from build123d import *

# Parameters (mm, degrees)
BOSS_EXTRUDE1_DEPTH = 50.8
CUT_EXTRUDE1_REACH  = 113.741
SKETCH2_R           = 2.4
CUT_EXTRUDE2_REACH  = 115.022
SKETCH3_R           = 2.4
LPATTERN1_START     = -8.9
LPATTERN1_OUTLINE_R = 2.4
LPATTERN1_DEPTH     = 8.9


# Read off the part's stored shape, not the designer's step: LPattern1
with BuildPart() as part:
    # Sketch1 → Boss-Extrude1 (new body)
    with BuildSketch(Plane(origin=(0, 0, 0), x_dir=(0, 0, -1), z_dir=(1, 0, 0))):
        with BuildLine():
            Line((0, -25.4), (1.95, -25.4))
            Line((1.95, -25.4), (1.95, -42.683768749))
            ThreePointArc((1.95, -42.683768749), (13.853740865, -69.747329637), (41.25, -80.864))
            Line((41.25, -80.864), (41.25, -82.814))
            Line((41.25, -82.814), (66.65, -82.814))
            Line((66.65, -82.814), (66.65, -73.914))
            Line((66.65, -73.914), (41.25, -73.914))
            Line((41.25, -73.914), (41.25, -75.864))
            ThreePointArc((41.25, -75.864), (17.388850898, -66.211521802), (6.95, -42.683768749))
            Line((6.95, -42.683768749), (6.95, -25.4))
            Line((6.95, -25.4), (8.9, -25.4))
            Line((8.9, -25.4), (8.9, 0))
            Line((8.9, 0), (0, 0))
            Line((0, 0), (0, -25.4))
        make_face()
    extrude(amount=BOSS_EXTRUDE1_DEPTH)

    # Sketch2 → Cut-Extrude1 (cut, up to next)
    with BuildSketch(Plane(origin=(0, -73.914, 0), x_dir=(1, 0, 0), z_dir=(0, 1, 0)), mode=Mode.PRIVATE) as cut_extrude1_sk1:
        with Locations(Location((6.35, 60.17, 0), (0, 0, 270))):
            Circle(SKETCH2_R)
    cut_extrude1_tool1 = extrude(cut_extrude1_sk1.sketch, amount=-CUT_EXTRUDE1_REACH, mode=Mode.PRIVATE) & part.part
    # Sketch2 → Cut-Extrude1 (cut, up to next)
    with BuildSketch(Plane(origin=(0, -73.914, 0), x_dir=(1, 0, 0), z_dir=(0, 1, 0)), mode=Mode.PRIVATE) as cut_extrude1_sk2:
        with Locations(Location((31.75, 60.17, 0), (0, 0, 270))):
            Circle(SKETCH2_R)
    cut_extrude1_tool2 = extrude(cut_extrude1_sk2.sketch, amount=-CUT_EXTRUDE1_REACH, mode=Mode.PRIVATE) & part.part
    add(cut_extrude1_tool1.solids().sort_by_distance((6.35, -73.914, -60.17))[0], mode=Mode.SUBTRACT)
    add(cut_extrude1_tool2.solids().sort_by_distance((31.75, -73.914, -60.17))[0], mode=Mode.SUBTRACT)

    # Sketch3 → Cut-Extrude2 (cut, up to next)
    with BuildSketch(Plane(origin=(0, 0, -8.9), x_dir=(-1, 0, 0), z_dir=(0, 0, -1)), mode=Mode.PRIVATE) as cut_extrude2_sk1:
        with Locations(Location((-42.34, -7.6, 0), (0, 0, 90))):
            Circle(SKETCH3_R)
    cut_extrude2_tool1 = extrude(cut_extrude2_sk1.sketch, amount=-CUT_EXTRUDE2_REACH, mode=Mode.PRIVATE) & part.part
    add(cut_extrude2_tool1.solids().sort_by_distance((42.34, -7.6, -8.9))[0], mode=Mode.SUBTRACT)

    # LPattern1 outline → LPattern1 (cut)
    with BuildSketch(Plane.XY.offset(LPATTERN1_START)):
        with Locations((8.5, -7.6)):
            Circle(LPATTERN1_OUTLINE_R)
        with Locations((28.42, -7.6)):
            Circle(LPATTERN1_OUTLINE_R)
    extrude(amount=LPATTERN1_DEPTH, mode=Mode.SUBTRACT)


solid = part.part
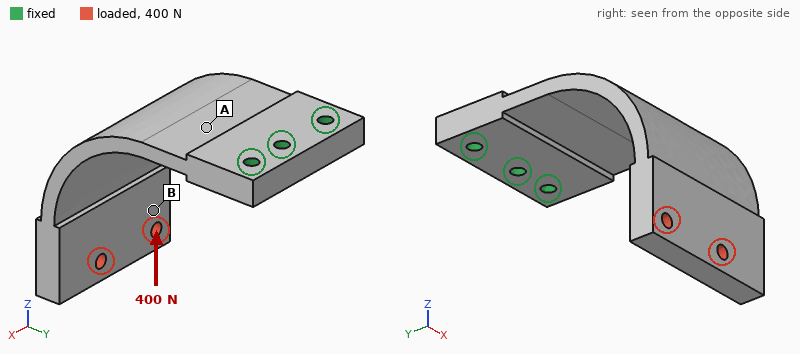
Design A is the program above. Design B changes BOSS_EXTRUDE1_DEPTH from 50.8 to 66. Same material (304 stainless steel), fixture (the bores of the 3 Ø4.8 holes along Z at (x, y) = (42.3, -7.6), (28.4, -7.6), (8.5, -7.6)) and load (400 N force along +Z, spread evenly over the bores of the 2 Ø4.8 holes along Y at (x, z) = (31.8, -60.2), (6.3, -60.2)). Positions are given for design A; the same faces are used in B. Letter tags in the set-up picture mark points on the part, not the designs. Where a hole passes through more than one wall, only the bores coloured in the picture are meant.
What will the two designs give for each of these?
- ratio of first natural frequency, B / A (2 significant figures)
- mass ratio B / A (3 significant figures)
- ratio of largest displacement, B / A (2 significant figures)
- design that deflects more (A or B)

0.99
1.31
0.81
A
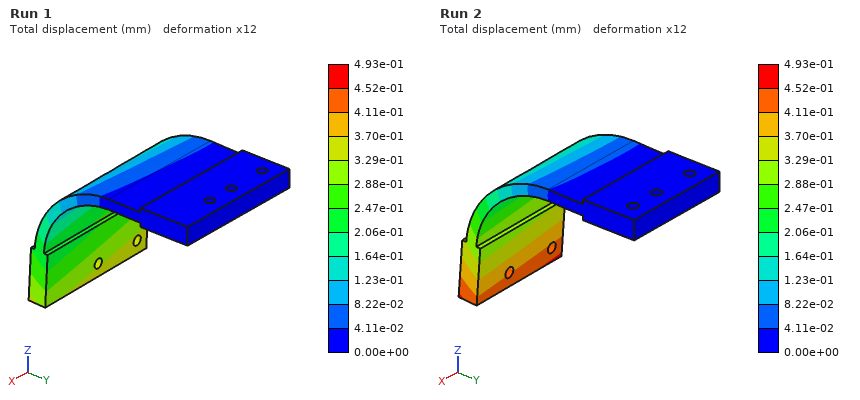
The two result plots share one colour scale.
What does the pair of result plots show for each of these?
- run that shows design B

Run 1
